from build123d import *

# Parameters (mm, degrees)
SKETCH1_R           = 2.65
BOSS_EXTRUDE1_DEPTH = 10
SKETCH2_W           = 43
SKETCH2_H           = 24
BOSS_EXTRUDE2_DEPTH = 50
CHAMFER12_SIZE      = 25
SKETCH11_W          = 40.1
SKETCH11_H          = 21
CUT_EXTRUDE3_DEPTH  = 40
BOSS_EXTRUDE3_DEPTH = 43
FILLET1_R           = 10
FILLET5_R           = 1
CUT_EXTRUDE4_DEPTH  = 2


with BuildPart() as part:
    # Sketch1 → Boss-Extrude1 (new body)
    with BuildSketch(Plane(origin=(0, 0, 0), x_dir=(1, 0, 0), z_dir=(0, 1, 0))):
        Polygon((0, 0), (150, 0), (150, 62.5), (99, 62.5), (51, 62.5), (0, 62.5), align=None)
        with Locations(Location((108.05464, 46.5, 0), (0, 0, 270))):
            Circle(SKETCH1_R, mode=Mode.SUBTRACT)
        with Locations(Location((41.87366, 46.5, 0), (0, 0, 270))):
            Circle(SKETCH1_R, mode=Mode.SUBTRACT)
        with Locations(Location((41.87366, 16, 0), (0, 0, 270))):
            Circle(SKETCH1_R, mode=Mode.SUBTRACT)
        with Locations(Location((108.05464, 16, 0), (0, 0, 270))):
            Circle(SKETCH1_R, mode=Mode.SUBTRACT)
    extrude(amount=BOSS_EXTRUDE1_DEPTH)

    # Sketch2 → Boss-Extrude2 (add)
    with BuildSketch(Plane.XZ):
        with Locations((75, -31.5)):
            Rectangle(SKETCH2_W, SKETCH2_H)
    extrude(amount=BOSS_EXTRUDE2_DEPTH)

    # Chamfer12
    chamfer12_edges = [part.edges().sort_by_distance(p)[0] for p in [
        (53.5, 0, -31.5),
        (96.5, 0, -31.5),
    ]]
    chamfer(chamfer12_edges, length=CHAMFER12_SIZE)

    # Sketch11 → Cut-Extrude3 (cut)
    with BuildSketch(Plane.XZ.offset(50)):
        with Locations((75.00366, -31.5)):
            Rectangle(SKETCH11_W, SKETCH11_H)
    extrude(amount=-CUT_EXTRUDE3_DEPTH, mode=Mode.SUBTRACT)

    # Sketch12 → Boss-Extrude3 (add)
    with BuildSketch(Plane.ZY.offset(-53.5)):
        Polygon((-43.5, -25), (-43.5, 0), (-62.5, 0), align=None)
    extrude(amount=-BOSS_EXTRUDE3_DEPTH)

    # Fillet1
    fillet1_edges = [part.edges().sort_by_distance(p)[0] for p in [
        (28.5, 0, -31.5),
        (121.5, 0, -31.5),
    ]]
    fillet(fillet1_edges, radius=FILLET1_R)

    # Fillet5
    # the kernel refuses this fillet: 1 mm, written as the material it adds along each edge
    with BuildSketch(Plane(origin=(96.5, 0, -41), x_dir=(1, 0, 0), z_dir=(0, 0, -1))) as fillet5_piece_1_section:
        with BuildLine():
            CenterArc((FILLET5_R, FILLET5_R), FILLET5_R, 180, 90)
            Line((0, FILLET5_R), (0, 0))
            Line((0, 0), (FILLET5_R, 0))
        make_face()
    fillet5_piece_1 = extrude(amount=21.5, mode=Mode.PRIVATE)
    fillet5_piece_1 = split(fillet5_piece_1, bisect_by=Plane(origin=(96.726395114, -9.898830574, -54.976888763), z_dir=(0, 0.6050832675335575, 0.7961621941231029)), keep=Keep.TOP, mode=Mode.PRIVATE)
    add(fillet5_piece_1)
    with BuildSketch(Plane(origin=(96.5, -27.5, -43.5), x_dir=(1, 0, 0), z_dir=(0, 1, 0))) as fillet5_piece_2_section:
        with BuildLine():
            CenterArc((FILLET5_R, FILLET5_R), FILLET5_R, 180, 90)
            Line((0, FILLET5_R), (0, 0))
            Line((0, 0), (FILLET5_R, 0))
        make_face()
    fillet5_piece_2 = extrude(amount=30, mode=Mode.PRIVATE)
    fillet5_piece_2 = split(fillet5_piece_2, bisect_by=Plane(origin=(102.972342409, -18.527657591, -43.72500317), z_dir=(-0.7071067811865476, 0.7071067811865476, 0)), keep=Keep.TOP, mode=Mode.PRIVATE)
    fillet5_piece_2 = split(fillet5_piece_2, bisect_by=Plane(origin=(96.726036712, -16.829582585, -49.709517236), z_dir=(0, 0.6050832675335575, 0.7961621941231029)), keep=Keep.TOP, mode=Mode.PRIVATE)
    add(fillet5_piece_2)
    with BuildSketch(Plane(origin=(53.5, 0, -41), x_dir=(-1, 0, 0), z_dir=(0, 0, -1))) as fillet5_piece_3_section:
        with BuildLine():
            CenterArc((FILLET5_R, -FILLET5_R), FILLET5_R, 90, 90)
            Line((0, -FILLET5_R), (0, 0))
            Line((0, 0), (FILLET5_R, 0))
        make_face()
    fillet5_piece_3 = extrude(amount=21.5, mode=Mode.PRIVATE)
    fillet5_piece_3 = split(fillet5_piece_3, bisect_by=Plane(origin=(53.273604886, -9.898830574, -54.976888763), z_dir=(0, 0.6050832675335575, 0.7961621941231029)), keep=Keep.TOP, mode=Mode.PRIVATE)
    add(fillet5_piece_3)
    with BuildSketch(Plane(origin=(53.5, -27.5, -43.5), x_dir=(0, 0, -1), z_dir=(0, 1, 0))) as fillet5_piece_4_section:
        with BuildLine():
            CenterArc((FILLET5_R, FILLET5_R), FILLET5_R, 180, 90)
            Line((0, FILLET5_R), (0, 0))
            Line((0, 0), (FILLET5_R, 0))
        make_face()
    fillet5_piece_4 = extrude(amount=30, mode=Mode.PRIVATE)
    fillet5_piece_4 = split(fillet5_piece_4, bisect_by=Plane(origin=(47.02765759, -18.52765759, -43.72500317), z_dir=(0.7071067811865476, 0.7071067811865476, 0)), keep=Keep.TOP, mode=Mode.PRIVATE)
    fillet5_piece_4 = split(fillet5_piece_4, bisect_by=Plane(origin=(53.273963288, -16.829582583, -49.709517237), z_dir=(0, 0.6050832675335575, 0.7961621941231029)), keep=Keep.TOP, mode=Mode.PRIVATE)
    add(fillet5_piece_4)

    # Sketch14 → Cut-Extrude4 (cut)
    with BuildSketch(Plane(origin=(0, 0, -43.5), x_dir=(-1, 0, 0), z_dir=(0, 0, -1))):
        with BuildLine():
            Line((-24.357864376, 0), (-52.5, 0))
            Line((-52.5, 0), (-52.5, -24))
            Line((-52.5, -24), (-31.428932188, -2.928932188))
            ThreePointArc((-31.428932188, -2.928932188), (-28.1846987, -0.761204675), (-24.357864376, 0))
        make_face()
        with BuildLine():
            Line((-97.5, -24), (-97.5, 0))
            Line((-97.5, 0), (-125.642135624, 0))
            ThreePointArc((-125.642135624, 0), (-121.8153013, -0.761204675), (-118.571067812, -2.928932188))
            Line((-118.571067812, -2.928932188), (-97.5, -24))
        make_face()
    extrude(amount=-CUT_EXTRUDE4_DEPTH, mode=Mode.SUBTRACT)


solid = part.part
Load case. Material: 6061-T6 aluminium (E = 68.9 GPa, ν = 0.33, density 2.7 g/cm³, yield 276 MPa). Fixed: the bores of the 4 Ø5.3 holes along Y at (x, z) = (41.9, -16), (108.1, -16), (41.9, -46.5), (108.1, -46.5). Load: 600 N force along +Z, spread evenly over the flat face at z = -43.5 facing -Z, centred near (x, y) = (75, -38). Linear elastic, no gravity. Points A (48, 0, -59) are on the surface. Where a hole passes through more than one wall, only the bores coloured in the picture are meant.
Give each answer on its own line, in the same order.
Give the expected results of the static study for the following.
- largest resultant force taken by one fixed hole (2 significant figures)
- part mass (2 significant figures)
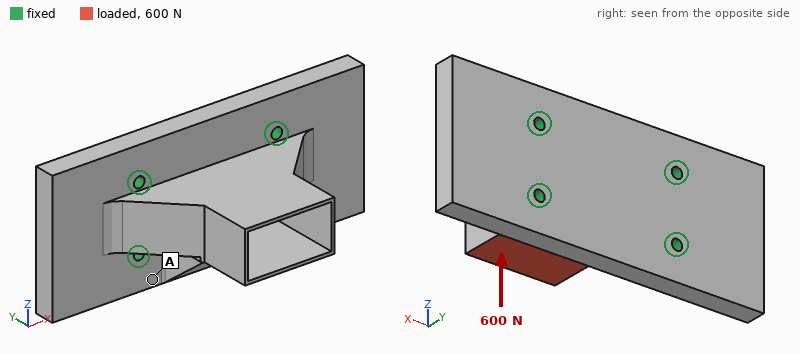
440 N
360 g
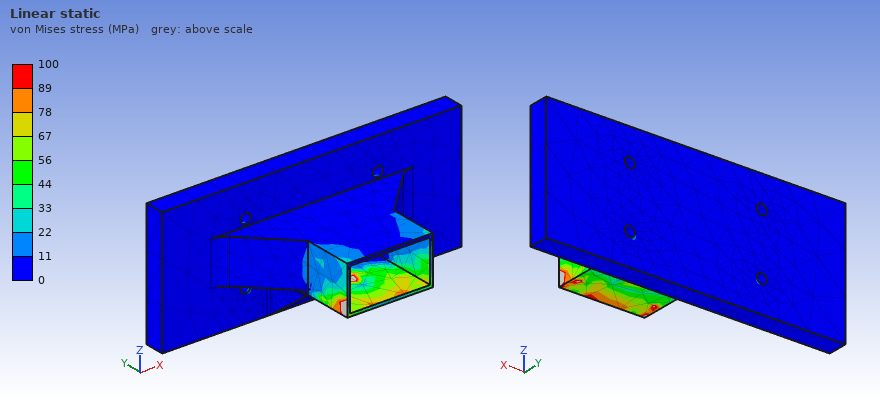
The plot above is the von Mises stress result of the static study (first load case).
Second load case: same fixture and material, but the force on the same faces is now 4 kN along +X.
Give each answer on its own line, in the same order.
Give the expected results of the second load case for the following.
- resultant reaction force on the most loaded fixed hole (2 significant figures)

2.2 kN
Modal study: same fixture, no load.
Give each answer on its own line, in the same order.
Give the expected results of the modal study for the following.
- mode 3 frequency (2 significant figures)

5100 Hz
